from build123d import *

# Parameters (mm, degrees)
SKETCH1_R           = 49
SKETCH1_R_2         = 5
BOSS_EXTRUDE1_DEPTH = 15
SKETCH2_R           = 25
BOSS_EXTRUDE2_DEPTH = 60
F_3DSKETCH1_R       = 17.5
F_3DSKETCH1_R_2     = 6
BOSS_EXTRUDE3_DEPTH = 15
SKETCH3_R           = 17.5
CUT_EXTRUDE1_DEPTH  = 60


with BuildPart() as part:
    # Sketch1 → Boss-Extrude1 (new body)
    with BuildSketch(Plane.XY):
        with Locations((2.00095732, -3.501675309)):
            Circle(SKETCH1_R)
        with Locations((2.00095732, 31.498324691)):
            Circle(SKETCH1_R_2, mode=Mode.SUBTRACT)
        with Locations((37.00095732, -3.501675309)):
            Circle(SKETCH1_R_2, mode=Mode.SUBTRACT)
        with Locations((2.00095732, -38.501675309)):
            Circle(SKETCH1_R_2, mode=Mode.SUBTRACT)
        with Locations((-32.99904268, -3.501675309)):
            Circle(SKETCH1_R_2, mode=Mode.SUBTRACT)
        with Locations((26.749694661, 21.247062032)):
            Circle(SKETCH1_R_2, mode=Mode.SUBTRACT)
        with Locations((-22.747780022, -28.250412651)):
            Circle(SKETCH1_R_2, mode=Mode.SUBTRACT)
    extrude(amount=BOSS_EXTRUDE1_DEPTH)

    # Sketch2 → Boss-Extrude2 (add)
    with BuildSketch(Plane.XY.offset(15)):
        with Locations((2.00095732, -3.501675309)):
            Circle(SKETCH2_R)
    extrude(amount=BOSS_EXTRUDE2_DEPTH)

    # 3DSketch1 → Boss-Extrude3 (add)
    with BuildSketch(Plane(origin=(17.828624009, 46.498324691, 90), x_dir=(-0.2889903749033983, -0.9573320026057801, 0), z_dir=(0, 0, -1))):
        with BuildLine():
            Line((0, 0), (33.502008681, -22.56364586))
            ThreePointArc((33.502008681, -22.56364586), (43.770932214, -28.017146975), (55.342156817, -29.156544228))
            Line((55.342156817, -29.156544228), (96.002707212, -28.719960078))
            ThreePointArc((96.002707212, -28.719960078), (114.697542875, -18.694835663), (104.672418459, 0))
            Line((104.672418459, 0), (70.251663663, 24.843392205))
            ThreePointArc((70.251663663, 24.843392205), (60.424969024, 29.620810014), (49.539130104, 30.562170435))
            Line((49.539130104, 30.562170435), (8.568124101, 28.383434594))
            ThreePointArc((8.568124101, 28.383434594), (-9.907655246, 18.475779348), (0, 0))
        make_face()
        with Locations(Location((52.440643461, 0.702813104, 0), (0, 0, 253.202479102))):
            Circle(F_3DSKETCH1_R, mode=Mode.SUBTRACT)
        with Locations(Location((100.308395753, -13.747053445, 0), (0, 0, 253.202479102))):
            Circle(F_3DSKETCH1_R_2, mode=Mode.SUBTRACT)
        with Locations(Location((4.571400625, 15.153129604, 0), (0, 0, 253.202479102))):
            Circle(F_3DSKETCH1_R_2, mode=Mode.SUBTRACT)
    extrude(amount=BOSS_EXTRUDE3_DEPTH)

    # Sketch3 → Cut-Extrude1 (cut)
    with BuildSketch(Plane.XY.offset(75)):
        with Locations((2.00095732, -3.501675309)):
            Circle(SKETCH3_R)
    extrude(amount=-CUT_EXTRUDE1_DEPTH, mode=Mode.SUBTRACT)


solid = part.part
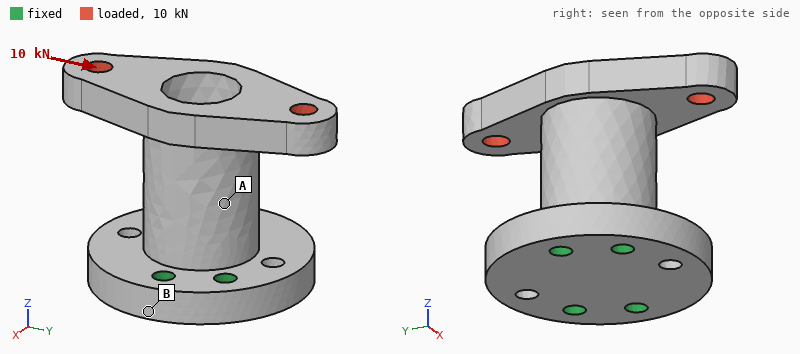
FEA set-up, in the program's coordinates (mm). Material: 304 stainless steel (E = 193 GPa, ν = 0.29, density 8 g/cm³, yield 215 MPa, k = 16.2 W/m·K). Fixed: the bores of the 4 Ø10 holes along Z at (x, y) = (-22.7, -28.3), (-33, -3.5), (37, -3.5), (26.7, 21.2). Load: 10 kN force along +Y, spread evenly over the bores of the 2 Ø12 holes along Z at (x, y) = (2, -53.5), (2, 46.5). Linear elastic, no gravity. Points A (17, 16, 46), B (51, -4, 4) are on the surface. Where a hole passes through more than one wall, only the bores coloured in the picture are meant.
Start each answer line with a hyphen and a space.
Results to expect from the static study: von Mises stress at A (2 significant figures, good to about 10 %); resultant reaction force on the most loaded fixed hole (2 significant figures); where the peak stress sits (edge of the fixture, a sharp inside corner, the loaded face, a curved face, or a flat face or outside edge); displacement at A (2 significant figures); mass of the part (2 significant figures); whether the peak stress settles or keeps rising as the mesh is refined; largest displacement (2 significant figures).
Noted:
- 35 MPa
- 12 kN
- edge of the fixture
- 0.035 mm
- 1.8 kg
- keeps rising
- 0.11 mm
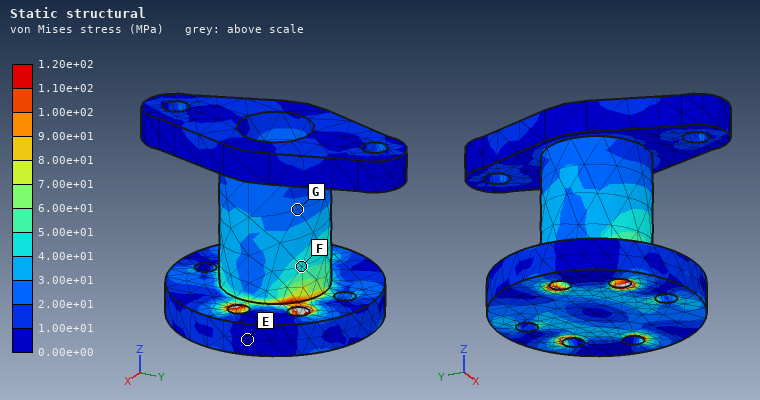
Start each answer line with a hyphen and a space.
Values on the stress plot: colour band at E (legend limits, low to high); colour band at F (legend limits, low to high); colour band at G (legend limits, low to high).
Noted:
- 0.00e+00 to 1.00e+01 MPa
- 4.00e+01 to 5.00e+01 MPa
- 2.00e+01 to 3.00e+01 MPa
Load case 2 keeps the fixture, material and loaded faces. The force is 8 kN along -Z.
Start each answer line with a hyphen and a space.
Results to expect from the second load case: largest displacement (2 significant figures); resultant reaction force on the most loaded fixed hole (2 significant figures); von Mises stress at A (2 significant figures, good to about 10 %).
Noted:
- 72 µm
- 2.3 kN
- 9.3 MPa
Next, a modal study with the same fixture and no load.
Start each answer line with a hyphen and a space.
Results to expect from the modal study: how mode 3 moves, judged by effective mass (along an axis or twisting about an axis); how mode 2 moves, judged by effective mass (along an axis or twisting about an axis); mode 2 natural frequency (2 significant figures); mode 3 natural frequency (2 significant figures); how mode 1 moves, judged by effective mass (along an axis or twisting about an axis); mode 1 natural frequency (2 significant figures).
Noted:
- twisting about Z
- along X
- 2700 Hz
- 4000 Hz
- along Y
- 2100 Hz
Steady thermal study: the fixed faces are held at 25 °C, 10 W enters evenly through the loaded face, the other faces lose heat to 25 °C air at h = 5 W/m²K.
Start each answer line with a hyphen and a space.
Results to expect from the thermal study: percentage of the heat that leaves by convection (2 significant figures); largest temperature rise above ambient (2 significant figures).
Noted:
- 39 %
- 51 K
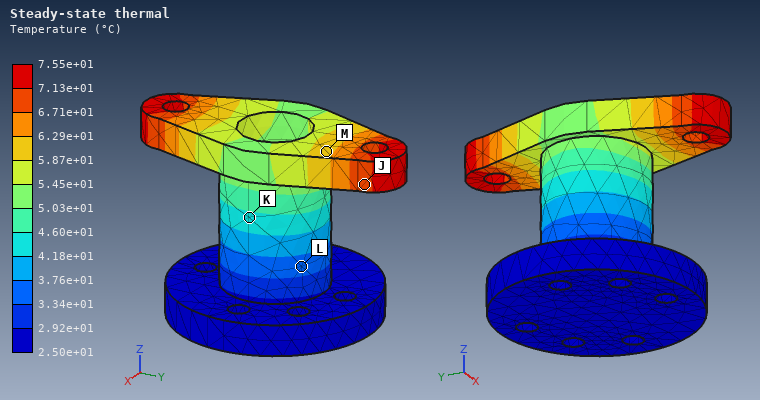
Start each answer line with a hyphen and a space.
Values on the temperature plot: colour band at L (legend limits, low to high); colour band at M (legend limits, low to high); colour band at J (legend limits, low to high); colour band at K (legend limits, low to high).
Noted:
- 3.34e+01 to 3.76e+01 °C
- 5.87e+01 to 6.29e+01 °C
- 6.71e+01 to 7.13e+01 °C
- 4.18e+01 to 4.60e+01 °C
